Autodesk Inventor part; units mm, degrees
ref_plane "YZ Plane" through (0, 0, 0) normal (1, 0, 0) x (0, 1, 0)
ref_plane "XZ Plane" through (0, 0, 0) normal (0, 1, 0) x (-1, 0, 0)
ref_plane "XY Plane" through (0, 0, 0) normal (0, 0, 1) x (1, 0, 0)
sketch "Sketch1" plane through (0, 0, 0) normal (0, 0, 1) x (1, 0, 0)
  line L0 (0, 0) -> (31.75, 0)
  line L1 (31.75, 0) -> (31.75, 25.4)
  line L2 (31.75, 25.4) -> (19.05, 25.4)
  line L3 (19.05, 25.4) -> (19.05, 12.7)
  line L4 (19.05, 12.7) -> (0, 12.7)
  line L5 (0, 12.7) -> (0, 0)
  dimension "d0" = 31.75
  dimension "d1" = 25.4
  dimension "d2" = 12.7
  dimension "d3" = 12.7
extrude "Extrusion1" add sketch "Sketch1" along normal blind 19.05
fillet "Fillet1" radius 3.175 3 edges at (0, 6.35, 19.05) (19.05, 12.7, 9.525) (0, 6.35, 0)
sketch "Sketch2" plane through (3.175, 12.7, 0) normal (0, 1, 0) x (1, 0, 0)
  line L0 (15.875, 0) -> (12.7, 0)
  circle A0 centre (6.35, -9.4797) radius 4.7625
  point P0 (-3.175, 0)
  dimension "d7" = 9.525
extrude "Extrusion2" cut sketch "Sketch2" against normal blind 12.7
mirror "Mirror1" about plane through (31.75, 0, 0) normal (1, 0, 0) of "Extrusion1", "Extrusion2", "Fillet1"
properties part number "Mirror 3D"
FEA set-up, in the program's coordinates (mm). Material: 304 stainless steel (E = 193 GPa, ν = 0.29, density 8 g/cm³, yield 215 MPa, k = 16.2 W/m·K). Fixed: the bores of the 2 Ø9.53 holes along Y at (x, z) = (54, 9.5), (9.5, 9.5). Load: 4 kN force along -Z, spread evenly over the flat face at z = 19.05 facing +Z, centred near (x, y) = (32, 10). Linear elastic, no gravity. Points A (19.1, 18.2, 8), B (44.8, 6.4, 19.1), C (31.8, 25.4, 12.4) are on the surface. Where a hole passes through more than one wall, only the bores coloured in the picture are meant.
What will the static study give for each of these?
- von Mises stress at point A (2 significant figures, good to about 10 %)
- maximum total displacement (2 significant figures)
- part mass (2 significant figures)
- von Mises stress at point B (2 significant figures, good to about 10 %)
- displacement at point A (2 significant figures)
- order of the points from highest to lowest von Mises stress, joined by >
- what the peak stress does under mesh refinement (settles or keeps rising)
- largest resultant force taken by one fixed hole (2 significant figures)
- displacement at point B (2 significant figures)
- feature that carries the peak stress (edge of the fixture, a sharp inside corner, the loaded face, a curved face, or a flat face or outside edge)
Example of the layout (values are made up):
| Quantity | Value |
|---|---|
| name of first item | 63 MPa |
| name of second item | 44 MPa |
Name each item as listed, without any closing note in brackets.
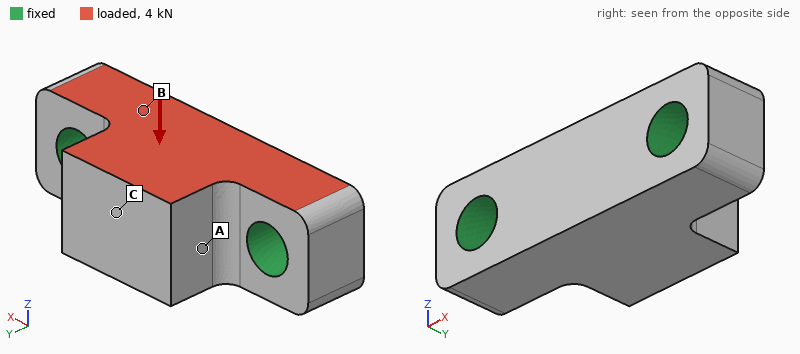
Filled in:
| Quantity | Value |
|---|---|
| von Mises stress at point A | 8.6 MPa |
| maximum total displacement | 4.3 µm |
| part mass | 160 g |
| von Mises stress at point B | 14 MPa |
| displacement at point A | 2.6 µm |
| order of the points from highest to lowest von Mises stress, joined by > | B > A > C |
| what the peak stress does under mesh refinement | keeps rising |
| largest resultant force taken by one fixed hole | 2.0 kN |
| displacement at point B | 1.2 µm |
| feature that carries the peak stress | edge of the fixture |
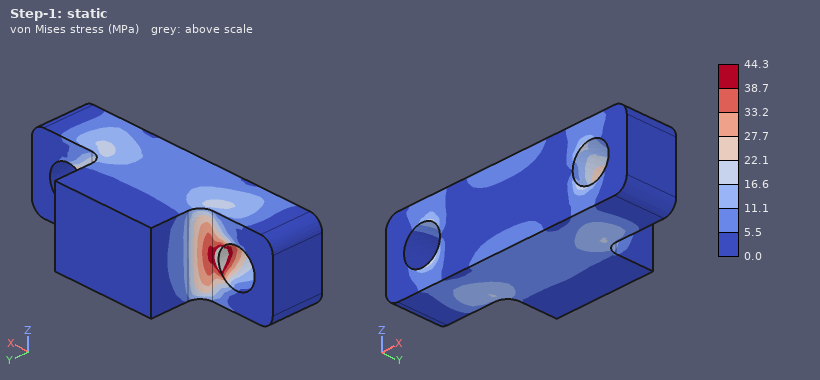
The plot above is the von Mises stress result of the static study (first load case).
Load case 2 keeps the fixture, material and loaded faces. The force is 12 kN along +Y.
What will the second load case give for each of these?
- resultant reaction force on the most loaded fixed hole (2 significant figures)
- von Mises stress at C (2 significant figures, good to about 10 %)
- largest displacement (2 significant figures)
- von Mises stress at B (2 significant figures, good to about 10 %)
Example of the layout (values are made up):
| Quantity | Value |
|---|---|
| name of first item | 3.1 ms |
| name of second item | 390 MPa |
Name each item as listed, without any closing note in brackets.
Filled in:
| Quantity | Value |
|---|---|
| resultant reaction force on the most loaded fixed hole | 6.1 kN |
| von Mises stress at C | 18 MPa |
| largest displacement | 17 µm |
| von Mises stress at B | 87 MPa |
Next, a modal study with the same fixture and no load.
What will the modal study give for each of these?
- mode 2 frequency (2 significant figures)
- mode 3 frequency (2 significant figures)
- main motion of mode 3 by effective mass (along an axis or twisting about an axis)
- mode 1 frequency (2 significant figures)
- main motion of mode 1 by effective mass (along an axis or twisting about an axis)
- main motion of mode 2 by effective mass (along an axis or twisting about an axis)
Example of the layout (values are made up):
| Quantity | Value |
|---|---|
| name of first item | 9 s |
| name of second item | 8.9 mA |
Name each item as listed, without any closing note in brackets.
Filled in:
| Quantity | Value |
|---|---|
| mode 2 frequency | 24 kHz |
| mode 3 frequency | 30 kHz |
| main motion of mode 3 by effective mass | along Z |
| mode 1 frequency | 14 kHz |
| main motion of mode 1 by effective mass | along Z |
| main motion of mode 2 by effective mass | along Y |
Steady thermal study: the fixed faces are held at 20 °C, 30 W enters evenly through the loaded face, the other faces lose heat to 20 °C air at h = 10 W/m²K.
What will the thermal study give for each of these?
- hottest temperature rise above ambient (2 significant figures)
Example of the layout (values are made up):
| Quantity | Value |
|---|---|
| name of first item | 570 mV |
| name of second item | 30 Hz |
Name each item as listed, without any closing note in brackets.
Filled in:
| Quantity | Value |
|---|---|
| hottest temperature rise above ambient | 47 K |
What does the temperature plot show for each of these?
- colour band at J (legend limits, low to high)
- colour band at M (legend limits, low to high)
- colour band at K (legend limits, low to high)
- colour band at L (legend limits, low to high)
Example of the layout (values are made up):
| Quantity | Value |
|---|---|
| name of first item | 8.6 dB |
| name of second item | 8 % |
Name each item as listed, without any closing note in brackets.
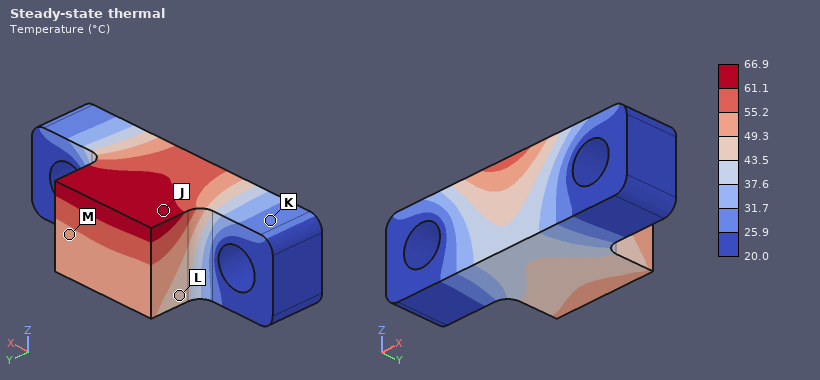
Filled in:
| Quantity | Value |
|---|---|
| colour band at J | 61.1 to 66.9 °C |
| colour band at M | 49.3 to 55.2 °C |
| colour band at K | 25.9 to 31.7 °C |
| colour band at L | 43.5 to 49.3 °C |
